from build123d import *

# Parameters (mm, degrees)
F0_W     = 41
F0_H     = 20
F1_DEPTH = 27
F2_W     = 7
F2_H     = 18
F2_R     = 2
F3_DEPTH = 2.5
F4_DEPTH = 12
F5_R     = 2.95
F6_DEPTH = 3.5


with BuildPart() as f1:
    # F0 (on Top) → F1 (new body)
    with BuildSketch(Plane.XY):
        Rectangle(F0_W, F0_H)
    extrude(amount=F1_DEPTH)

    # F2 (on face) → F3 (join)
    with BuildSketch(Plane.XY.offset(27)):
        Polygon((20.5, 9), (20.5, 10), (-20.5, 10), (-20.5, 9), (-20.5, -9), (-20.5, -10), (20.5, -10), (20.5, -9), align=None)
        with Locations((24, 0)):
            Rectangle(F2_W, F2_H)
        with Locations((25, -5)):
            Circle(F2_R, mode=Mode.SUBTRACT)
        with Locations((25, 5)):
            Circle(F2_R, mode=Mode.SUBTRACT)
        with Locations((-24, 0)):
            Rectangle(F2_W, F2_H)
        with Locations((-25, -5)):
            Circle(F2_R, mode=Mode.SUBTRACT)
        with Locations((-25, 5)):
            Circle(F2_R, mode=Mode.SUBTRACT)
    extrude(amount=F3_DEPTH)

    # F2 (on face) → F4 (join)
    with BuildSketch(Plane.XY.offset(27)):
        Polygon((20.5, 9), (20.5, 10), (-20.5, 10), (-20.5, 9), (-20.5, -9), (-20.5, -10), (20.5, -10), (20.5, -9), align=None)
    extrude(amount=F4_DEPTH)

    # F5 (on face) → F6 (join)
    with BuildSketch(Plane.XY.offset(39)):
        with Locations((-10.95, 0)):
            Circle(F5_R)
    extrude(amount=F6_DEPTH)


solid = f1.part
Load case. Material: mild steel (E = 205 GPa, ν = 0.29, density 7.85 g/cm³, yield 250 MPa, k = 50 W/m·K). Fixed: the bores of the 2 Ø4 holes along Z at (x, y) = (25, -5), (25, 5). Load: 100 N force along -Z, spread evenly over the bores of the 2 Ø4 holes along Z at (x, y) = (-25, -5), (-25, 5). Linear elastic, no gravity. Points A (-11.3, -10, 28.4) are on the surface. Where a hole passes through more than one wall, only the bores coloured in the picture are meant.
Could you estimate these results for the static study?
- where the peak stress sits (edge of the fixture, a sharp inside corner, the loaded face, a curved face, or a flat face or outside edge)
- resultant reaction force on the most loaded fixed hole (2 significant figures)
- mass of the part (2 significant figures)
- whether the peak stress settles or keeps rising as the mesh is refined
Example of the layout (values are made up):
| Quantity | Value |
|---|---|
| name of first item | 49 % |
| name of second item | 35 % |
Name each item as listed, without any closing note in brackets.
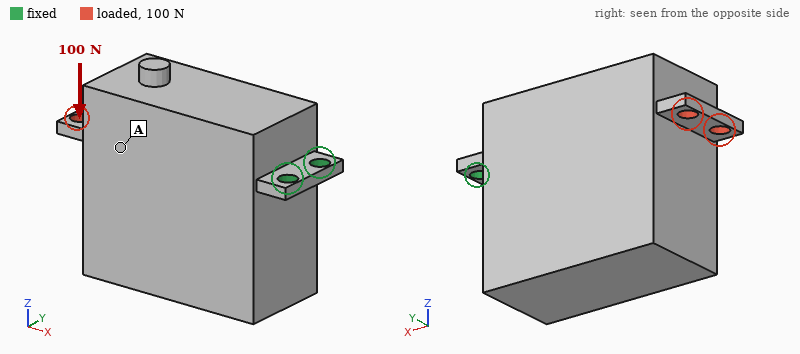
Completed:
| Quantity | Value |
|---|---|
| where the peak stress sits | edge of the fixture |
| resultant reaction force on the most loaded fixed hole | 51 N |
| mass of the part | 260 g |
| whether the peak stress settles or keeps rising as the mesh is refined | keeps rising |
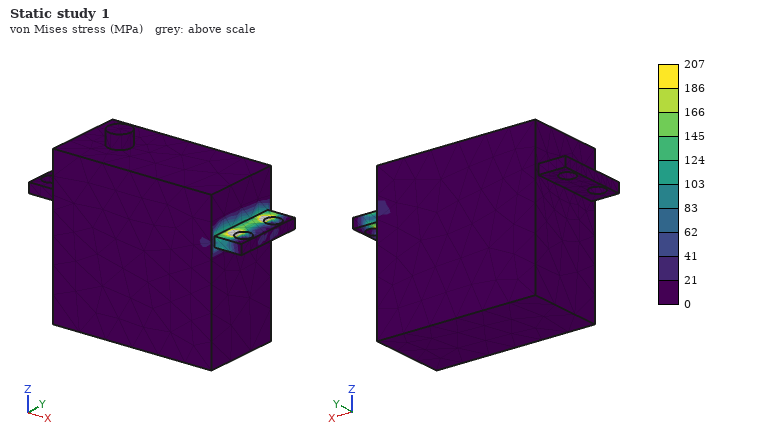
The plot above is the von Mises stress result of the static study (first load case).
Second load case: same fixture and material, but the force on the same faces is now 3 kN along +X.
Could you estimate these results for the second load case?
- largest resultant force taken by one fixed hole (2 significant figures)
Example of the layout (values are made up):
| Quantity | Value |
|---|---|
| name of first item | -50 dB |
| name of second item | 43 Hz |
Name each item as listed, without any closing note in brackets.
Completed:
| Quantity | Value |
|---|---|
| largest resultant force taken by one fixed hole | 1.5 kN |
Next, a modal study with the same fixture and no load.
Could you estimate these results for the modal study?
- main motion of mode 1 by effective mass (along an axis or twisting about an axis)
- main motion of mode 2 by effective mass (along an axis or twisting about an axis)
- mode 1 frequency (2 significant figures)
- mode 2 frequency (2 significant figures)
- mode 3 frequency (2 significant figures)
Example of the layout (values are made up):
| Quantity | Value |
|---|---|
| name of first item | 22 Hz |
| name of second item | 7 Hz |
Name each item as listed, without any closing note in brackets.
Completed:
| Quantity | Value |
|---|---|
| main motion of mode 1 by effective mass | along Z |
| main motion of mode 2 by effective mass | along Y |
| mode 1 frequency | 390 Hz |
| mode 2 frequency | 1900 Hz |
| mode 3 frequency | 3100 Hz |
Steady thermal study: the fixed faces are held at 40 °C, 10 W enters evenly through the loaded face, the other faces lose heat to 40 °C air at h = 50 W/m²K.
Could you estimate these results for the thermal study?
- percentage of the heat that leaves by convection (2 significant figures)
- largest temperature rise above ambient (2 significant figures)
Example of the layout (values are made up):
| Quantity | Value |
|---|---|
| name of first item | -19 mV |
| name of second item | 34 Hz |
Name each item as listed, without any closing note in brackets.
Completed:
| Quantity | Value |
|---|---|
| percentage of the heat that leaves by convection | 52 % |
| largest temperature rise above ambient | 61 K |
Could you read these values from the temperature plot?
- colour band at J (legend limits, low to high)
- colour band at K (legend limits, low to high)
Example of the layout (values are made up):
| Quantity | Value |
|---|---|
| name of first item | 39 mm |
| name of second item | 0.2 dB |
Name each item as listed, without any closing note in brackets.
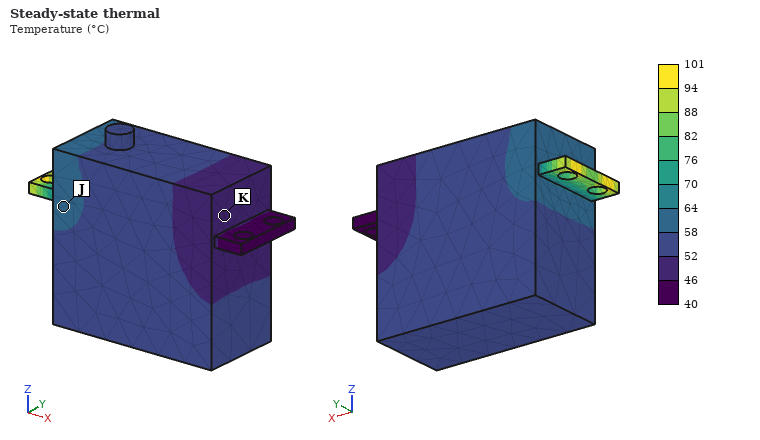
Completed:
| Quantity | Value |
|---|---|
| colour band at J | 58 to 64 °C |
| colour band at K | 46 to 52 °C |
